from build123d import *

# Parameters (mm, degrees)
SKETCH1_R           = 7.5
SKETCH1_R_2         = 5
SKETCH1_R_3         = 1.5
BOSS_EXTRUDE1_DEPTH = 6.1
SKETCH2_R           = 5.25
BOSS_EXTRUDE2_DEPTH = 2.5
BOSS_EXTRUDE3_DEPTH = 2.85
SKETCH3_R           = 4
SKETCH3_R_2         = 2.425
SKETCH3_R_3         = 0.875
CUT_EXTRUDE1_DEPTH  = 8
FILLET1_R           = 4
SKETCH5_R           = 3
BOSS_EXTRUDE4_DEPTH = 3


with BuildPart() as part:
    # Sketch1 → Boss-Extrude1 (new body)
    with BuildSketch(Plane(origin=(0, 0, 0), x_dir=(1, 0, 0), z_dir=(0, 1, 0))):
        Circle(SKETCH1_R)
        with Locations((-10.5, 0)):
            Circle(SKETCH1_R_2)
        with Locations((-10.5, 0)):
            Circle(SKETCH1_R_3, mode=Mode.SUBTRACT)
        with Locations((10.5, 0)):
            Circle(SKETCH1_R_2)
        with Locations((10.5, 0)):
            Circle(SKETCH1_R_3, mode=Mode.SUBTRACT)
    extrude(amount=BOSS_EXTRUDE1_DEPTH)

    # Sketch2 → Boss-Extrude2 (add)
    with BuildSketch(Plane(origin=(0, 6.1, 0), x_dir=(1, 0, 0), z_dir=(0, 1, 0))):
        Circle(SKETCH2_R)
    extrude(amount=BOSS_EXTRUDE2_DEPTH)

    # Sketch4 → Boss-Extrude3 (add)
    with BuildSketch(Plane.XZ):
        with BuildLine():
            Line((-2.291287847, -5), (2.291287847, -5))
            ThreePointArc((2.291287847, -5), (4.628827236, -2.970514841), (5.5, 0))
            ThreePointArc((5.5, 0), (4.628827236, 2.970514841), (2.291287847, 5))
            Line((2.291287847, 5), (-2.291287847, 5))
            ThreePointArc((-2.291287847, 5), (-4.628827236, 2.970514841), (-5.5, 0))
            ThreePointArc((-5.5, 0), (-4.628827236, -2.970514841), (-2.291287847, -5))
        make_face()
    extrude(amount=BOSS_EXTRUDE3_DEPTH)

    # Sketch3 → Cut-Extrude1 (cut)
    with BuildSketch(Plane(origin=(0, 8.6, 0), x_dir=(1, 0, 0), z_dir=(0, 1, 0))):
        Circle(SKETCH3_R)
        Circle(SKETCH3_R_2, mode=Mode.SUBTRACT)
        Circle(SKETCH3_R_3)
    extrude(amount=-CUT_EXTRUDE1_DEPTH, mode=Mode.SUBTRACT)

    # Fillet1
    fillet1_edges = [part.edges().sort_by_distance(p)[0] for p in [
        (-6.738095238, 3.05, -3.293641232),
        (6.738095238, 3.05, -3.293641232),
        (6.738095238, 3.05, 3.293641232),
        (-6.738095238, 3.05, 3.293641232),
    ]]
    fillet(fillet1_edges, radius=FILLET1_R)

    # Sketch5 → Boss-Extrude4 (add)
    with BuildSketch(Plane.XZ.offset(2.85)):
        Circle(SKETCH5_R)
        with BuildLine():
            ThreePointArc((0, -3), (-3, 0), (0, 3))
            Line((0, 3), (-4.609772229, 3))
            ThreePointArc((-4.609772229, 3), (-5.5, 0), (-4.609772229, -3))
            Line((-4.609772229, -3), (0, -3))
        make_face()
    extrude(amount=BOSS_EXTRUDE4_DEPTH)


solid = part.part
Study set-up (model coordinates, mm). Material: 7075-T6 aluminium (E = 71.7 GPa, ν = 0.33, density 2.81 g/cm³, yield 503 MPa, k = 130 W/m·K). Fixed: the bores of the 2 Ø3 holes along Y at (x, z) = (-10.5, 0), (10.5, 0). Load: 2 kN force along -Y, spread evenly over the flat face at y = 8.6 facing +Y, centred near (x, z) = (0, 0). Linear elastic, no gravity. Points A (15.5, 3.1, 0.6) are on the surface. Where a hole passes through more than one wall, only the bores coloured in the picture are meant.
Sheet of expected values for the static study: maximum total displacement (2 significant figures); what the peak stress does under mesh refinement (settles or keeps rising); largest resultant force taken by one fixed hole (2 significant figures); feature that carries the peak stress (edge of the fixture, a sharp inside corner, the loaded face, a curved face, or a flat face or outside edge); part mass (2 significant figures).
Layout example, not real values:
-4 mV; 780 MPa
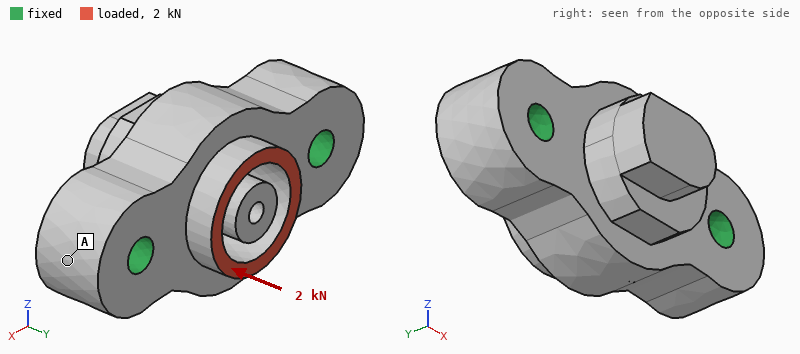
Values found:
13 µm; keeps rising; 1.0 kN; edge of the fixture; 6.2 g
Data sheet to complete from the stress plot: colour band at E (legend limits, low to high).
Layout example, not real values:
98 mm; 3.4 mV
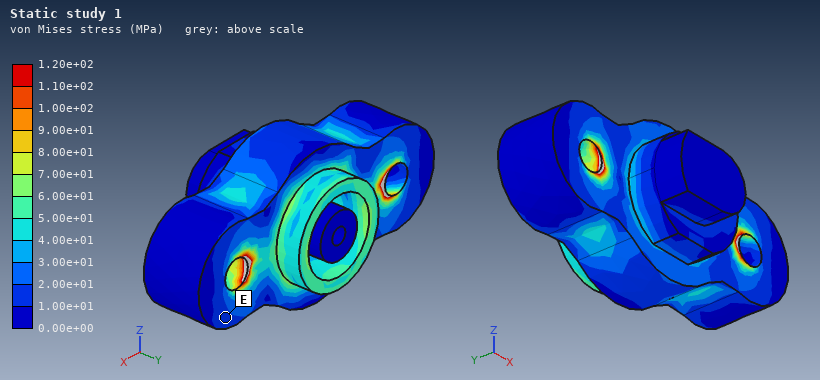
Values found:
1.00e+01 to 2.00e+01 MPa
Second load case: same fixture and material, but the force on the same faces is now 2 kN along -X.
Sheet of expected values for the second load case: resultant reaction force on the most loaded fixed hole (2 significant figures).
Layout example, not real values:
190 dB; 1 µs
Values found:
1.2 kN
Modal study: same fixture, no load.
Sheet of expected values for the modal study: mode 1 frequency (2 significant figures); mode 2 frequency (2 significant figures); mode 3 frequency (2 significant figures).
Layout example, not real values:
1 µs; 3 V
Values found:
30 kHz; 35 kHz; 36 kHz
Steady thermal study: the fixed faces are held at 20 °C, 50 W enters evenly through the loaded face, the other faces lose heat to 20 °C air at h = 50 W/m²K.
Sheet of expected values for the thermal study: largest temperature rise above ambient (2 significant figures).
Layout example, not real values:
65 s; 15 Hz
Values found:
59 K
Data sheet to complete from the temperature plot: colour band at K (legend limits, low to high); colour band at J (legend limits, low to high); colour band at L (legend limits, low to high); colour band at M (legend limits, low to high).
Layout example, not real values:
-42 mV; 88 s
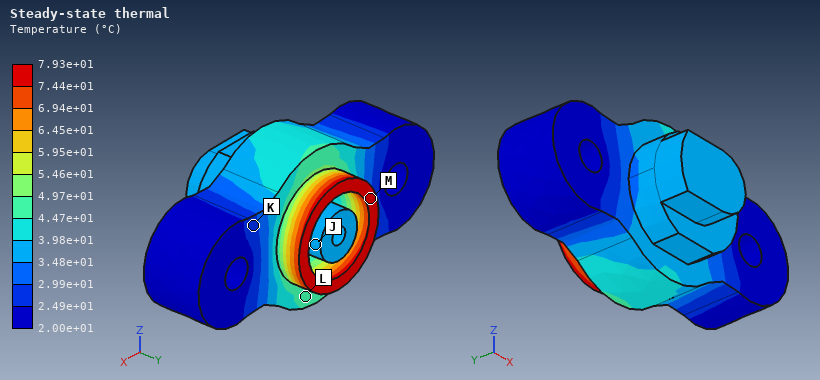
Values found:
2.49e+01 to 2.99e+01 °C; 3.48e+01 to 3.98e+01 °C; 4.47e+01 to 4.97e+01 °C; 7.44e+01 to 7.93e+01 °C
